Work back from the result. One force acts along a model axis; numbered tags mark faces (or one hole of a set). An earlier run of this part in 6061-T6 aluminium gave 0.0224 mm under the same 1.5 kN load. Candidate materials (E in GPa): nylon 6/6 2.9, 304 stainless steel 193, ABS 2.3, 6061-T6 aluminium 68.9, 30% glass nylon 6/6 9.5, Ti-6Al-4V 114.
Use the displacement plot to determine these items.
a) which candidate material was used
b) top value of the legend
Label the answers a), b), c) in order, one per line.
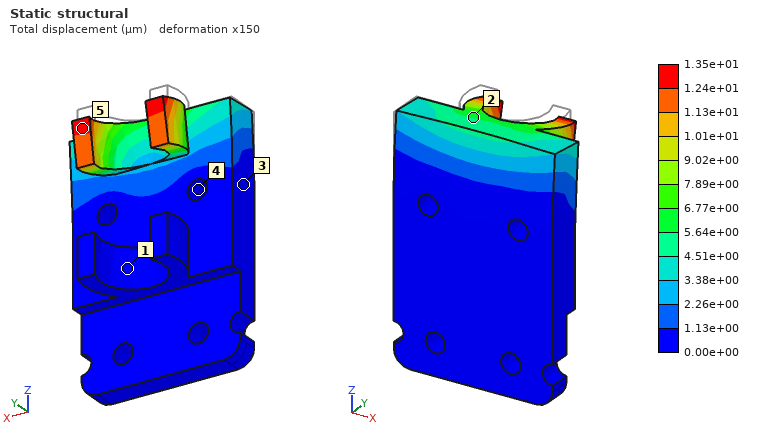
a) Ti-6Al-4V
b) 1.35e+01 µm
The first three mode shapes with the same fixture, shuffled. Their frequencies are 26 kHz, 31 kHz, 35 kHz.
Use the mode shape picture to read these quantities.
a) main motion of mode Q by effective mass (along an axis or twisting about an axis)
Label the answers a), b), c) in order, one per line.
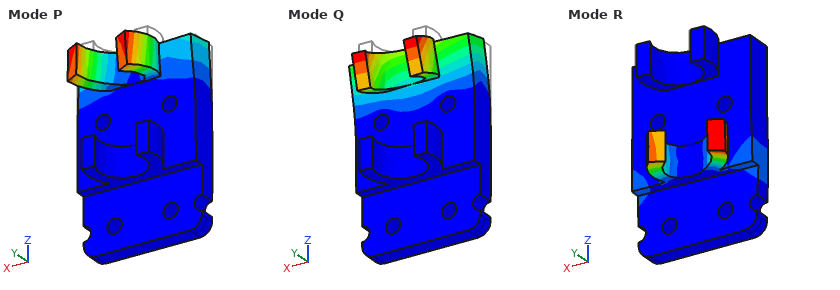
a) along Y
